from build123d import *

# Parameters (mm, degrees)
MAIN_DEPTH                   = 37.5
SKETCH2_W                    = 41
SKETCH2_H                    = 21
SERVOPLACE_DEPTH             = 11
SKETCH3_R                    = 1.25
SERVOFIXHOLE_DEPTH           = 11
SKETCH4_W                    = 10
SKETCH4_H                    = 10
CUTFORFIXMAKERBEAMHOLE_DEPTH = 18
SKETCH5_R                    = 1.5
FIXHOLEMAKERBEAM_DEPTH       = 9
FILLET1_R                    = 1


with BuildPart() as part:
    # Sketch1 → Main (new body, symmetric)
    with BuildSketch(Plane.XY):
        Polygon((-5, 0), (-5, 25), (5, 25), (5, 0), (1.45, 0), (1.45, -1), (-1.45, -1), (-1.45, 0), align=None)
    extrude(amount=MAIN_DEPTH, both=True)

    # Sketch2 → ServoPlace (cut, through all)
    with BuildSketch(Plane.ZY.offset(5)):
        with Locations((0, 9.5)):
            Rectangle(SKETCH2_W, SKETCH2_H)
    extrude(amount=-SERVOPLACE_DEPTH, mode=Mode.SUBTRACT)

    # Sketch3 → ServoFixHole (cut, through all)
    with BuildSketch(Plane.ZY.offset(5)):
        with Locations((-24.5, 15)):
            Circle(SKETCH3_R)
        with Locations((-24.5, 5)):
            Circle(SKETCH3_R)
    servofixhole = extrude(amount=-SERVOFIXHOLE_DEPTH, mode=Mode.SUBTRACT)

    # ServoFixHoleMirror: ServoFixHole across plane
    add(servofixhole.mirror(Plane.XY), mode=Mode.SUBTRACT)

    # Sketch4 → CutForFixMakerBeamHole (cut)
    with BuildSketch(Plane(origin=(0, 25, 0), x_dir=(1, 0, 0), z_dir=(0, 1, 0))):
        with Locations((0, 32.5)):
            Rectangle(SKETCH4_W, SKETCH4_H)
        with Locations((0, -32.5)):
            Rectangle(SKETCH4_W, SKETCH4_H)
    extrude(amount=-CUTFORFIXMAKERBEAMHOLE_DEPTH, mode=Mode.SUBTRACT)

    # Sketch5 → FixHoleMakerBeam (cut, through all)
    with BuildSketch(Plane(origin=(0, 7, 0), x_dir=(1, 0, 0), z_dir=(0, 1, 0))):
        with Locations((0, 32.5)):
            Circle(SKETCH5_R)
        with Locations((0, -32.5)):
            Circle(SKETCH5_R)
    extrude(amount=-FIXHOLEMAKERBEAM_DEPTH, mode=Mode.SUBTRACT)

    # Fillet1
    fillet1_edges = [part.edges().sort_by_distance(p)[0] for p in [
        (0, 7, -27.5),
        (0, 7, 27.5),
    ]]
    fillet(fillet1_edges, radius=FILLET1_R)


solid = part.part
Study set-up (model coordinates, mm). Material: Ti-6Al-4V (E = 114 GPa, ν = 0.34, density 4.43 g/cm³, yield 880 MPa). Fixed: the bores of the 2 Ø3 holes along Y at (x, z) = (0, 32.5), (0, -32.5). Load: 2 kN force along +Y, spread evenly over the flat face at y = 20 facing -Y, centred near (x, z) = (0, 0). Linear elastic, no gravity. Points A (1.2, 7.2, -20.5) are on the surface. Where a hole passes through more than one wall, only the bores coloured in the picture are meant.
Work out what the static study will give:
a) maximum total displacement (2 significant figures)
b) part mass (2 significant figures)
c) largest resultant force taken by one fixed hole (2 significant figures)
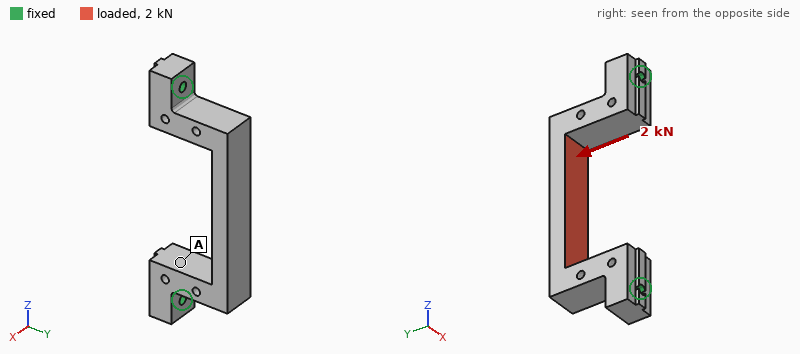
69 µm
30 g
1.2 kN
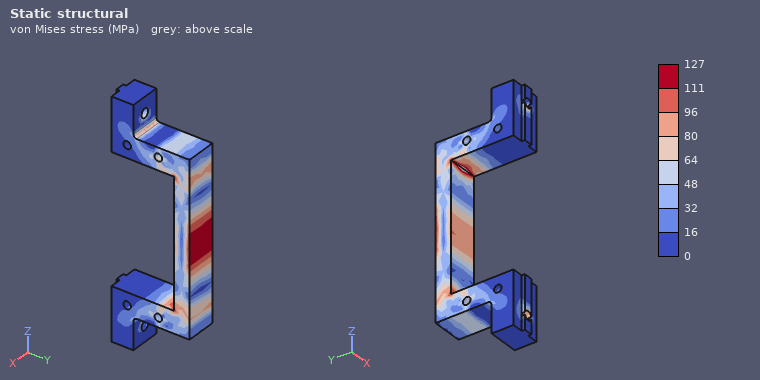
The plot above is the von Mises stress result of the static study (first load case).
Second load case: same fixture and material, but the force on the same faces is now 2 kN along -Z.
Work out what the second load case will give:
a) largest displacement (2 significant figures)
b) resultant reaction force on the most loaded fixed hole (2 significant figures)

81 µm
1.0 kN
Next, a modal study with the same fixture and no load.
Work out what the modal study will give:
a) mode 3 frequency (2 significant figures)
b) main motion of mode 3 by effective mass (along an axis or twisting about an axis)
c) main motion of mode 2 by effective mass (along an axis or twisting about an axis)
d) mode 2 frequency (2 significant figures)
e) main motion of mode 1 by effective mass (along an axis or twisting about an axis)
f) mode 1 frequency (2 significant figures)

8600 Hz
twisting about Y
along Z
6800 Hz
along X
4800 Hz
